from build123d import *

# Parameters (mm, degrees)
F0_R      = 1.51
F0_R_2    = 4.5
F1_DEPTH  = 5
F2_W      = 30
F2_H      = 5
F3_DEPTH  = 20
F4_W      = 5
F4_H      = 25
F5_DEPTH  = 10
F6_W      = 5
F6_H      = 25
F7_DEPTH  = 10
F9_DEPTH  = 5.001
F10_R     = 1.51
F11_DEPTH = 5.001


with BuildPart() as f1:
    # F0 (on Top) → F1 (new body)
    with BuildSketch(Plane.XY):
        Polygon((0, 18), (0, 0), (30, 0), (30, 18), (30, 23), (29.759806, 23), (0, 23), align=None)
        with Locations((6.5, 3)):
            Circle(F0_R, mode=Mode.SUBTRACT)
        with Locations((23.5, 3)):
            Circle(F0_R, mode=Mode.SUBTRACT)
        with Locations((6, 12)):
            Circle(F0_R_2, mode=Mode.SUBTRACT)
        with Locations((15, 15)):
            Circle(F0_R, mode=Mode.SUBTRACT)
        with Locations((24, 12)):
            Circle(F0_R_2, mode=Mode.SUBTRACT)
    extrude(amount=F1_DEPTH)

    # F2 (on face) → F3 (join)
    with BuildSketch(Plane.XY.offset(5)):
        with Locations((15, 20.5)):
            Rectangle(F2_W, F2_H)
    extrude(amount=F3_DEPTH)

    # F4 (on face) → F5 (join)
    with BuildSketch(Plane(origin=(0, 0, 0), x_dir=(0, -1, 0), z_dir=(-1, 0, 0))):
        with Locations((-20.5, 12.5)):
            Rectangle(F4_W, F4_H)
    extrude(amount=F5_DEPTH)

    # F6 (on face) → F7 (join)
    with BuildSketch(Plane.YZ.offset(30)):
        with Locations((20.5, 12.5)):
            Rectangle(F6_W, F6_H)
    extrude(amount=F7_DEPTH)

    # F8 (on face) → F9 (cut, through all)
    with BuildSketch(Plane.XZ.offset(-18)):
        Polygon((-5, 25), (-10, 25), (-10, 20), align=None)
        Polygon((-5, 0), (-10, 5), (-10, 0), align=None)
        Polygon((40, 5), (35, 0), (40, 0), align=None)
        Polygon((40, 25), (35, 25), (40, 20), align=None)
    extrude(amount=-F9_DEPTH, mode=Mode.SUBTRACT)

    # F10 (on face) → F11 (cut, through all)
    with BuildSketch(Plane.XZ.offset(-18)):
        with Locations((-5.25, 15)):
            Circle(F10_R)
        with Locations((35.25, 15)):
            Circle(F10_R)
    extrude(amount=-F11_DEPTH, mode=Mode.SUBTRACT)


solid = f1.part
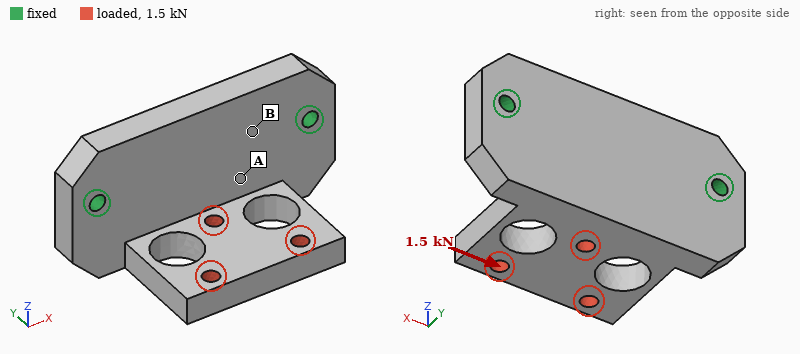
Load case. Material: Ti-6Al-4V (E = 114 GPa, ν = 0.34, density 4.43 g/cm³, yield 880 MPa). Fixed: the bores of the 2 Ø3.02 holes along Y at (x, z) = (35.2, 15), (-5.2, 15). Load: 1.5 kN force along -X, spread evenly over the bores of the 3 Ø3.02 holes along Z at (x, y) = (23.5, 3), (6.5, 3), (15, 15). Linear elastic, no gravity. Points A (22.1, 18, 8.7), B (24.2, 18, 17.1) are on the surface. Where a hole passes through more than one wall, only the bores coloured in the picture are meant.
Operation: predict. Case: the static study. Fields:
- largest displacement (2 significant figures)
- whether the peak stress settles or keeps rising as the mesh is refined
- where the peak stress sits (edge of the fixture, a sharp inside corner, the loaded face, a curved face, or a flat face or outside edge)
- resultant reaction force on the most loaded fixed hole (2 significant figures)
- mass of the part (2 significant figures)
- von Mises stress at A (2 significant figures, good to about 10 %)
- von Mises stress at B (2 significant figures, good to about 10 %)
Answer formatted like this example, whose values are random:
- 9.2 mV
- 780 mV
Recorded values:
- 49 µm
- keeps rising
- edge of the fixture
- 1.0 kN
- 35 g
- 50 MPa
- 21 MPa
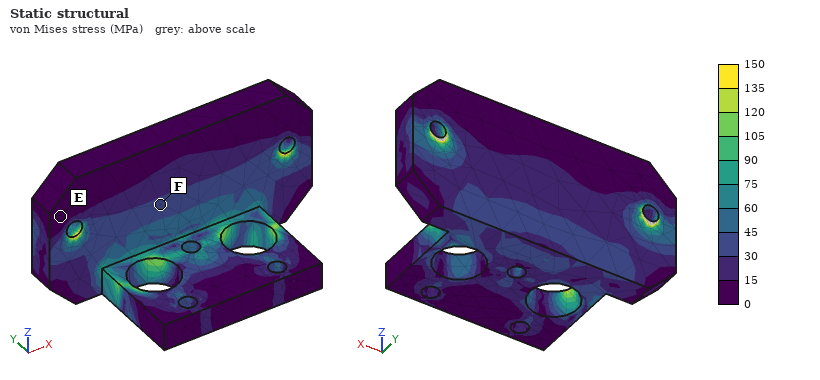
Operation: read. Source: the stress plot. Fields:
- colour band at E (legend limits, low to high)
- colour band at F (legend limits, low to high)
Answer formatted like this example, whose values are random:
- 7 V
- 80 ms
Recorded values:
- 0 to 15 MPa
- 30 to 45 MPa
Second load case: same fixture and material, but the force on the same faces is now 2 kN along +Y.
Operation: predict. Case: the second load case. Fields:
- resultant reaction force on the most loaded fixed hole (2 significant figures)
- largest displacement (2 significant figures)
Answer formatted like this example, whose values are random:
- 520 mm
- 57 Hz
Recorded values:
- 1.0 kN
- 0.13 mm
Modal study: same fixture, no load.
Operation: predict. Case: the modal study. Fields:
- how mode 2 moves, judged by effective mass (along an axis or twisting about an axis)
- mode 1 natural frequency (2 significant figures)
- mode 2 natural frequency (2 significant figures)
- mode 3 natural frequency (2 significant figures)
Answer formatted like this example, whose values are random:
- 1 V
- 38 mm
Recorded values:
- along Y
- 4700 Hz
- 9500 Hz
- 10000 Hz
